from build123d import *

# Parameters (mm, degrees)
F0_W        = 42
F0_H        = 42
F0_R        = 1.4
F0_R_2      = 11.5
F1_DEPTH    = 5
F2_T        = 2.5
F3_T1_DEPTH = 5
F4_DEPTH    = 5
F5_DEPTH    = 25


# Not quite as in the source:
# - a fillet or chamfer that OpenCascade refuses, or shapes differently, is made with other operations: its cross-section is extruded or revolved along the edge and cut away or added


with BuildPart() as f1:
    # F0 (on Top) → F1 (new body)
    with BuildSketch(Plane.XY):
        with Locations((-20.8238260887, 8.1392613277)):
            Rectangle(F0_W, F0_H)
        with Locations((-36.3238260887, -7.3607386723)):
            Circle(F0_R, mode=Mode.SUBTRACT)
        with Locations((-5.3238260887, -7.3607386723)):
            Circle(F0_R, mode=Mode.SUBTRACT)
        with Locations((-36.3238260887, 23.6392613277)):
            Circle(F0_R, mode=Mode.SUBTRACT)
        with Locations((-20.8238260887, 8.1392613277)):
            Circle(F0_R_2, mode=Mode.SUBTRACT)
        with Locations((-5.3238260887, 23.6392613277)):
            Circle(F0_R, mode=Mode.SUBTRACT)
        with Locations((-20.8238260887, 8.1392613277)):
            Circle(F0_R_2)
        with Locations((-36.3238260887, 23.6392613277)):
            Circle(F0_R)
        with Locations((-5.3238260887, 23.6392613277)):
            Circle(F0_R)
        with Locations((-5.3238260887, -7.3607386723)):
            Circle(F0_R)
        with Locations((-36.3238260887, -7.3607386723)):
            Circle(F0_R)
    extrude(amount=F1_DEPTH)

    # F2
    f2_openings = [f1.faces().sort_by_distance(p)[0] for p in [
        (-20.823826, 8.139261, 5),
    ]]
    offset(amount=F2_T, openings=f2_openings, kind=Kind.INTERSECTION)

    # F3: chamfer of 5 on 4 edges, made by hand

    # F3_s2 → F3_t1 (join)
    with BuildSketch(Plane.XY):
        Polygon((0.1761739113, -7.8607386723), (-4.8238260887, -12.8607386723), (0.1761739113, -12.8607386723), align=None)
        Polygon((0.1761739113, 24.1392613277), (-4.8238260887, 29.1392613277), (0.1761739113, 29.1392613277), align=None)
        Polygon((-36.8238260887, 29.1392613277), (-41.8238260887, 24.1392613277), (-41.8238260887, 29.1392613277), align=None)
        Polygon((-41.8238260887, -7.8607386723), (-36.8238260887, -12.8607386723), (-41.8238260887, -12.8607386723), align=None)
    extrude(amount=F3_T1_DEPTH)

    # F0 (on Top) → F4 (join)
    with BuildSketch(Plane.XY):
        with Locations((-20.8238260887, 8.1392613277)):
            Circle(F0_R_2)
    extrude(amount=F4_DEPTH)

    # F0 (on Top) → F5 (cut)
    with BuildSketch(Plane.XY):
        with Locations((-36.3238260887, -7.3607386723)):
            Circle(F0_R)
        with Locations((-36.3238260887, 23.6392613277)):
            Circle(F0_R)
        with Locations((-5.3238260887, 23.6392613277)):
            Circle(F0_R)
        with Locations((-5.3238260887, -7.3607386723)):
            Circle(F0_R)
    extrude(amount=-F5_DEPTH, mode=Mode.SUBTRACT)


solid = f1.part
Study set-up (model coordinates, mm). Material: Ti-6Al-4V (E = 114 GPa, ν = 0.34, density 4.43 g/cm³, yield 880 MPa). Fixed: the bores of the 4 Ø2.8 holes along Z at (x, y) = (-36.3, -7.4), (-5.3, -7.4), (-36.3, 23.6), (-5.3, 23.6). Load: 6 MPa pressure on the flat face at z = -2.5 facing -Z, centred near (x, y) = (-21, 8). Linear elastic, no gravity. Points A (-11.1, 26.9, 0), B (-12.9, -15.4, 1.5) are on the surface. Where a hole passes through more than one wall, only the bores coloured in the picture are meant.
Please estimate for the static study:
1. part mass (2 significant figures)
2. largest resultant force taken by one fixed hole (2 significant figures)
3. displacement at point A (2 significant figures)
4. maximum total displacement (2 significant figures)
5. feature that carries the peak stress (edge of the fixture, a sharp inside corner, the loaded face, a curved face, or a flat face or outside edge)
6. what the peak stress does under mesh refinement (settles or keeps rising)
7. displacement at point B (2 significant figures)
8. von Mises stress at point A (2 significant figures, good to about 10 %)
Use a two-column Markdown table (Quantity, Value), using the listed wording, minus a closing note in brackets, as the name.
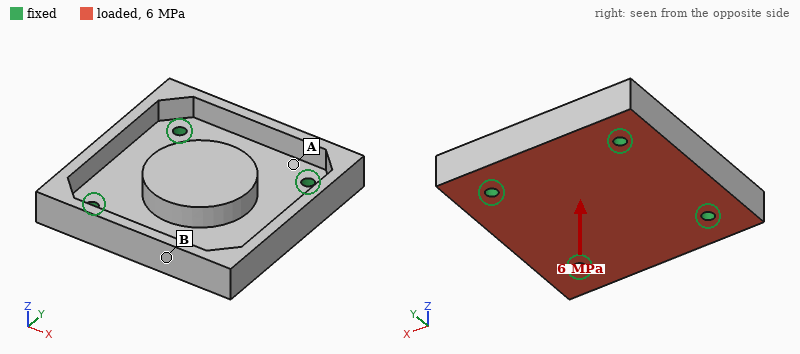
| Quantity | Value |
|---|---|
| part mass | 44 g |
| largest resultant force taken by one fixed hole | 3.3 kN |
| displacement at point A | 25 µm |
| maximum total displacement | 81 µm |
| feature that carries the peak stress | edge of the fixture |
| what the peak stress does under mesh refinement | keeps rising |
| displacement at point B | 23 µm |
| von Mises stress at point A | 140 MPa |
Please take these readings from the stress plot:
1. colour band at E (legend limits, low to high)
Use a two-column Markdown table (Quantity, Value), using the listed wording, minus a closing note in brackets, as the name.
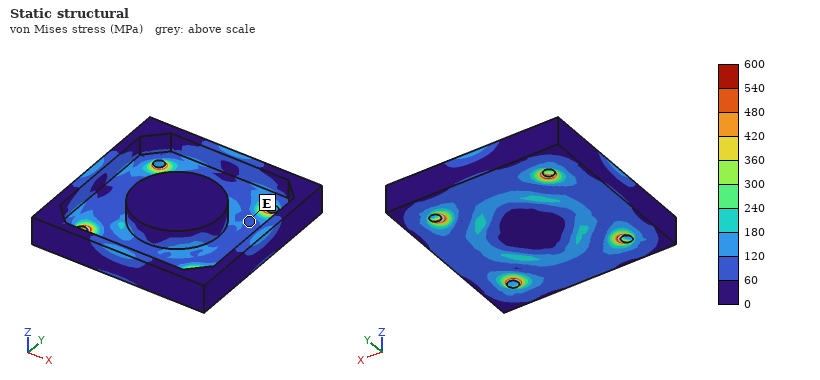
| Quantity | Value |
|---|---|
| colour band at E | 60 to 120 MPa |
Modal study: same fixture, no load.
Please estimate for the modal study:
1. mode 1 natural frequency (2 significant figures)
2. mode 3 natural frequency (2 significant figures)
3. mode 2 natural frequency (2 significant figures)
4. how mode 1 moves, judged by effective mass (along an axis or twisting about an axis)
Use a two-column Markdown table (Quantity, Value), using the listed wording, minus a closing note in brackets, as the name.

| Quantity | Value |
|---|---|
| mode 1 natural frequency | 10000 Hz |
| mode 3 natural frequency | 15 kHz |
| mode 2 natural frequency | 14 kHz |
| how mode 1 moves, judged by effective mass | along Z |
